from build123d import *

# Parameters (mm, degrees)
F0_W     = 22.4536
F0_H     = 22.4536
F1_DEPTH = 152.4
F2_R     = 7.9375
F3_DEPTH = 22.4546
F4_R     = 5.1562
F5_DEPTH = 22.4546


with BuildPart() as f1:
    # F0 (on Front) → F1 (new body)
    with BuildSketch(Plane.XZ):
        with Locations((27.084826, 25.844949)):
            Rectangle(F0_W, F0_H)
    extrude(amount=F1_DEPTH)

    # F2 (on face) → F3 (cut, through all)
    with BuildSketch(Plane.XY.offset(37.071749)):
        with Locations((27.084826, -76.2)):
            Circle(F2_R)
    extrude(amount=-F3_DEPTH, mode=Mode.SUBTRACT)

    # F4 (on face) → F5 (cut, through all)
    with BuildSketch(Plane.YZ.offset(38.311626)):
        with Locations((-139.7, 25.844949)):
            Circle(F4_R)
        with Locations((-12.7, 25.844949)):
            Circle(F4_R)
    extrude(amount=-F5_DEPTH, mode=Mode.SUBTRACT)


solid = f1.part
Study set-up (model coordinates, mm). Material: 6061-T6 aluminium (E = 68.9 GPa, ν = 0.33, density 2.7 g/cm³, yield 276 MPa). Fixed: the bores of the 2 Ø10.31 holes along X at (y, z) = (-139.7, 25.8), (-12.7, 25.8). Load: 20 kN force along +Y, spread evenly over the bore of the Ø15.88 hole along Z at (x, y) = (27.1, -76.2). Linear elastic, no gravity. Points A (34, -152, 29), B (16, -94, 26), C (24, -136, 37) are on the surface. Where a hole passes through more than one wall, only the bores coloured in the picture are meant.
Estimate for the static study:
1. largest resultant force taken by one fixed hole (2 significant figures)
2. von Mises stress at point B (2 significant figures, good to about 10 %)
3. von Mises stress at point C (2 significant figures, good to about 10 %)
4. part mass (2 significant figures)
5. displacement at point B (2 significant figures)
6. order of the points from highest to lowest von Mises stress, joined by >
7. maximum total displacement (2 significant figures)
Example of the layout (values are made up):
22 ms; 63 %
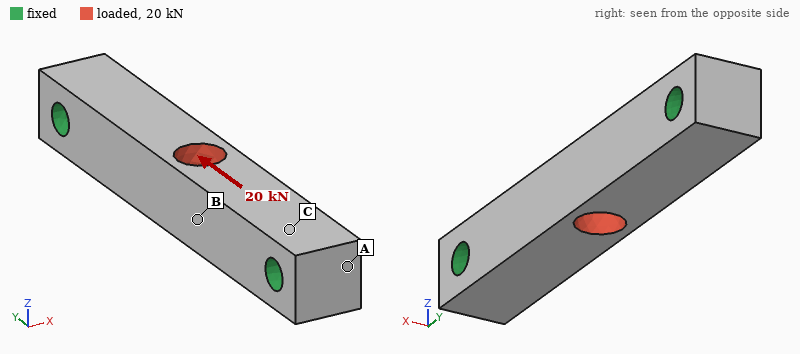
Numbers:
10 kN; 21 MPa; 9.8 MPa; 190 g; 13 µm; B > C > A; 18 µm
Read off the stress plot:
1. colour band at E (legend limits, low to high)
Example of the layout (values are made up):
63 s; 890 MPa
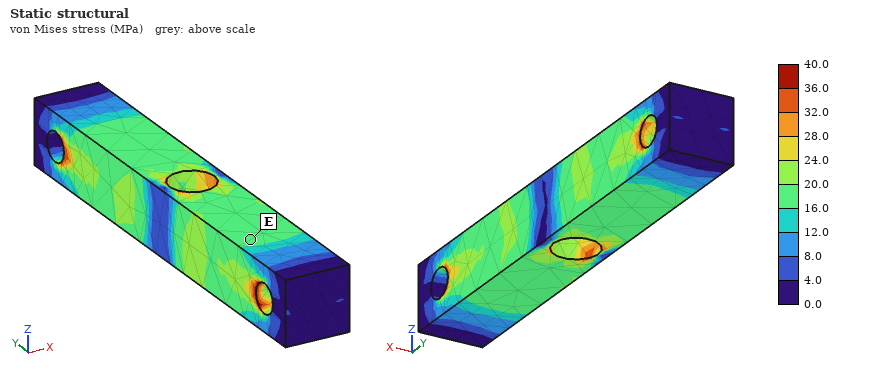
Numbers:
16.0 to 20.0 MPa
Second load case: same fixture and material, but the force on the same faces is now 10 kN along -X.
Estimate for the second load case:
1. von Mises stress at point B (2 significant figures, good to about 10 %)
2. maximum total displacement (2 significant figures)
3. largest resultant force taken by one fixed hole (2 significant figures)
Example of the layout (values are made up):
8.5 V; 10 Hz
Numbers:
31 MPa; 96 µm; 5.0 kN
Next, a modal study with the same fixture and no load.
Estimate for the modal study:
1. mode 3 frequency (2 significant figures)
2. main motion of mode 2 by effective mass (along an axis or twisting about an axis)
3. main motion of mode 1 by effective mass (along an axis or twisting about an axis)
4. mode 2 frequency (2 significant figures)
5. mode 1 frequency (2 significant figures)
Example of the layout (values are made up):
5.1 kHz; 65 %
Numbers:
12 kHz; along X; along Z; 7000 Hz; 5700 Hz
